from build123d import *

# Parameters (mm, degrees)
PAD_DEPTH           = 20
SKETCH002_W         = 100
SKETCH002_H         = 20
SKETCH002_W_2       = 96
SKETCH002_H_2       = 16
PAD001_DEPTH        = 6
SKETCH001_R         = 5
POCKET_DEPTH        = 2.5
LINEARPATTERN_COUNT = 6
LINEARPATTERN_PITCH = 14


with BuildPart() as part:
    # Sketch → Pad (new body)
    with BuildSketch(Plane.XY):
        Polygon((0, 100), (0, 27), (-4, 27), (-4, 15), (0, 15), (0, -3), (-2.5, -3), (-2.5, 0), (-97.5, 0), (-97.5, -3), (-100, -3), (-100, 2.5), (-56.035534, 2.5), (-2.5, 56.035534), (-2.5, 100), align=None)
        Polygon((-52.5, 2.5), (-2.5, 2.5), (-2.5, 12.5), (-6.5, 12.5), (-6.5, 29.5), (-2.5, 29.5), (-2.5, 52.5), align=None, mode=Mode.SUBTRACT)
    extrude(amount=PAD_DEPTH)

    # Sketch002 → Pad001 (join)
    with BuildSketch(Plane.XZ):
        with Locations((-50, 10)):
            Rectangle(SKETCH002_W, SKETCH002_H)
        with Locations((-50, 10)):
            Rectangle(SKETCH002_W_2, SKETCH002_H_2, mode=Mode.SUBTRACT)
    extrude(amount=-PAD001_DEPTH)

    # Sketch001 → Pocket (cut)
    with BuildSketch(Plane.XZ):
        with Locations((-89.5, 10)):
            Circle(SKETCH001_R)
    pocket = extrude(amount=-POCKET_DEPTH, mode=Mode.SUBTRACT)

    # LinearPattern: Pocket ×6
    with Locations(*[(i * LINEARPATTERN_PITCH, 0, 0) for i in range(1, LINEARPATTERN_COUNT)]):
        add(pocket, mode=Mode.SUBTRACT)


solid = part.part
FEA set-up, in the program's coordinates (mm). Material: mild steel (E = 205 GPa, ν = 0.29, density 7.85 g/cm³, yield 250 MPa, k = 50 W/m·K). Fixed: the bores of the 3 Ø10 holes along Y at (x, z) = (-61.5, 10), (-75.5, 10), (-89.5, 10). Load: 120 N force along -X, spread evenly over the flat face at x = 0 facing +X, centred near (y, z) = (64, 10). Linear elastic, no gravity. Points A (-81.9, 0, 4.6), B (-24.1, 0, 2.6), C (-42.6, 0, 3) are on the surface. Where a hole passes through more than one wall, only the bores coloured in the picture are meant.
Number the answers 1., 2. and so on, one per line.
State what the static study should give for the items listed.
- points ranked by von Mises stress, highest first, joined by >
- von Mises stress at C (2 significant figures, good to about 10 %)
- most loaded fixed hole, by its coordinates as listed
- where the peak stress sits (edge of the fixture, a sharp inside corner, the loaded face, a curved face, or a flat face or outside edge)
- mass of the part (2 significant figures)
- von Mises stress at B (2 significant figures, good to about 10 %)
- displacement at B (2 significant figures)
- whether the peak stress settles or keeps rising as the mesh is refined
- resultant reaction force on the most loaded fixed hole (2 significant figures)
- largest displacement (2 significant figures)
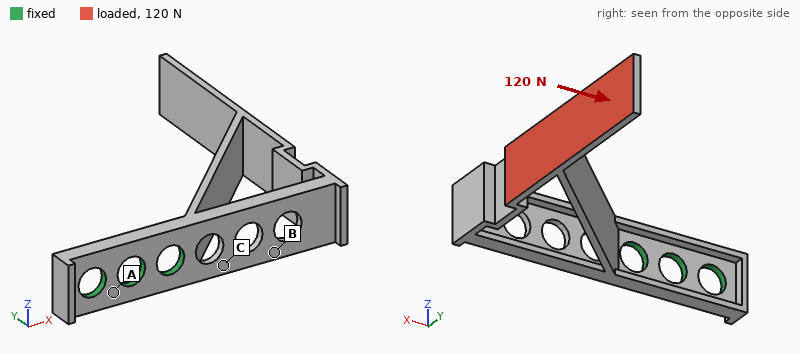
1. C > B > A
2. 89 MPa
3. (-75.5, 10)
4. edge of the fixture
5. 110 g
6. 42 MPa
7. 0.15 mm
8. keeps rising
9. 330 N
10. 0.88 mm
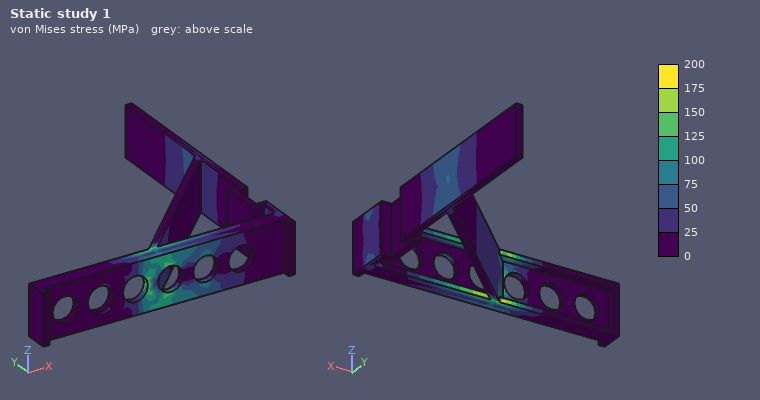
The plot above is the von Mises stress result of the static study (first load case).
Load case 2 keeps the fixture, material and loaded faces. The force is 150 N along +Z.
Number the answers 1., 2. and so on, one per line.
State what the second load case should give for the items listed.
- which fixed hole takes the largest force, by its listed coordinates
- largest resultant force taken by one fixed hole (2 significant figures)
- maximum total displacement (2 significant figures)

1. (-61.5, 10)
2. 250 N
3. 0.25 mm
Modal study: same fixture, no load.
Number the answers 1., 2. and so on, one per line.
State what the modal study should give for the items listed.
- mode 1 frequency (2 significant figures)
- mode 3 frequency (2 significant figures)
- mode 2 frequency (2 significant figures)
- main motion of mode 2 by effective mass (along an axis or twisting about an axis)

1. 320 Hz
2. 900 Hz
3. 800 Hz
4. along Z
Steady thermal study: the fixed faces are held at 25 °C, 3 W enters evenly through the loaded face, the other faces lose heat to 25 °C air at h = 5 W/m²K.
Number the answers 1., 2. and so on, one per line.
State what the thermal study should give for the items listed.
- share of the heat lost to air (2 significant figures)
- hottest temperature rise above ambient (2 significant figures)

1. 38 %
2. 53 K
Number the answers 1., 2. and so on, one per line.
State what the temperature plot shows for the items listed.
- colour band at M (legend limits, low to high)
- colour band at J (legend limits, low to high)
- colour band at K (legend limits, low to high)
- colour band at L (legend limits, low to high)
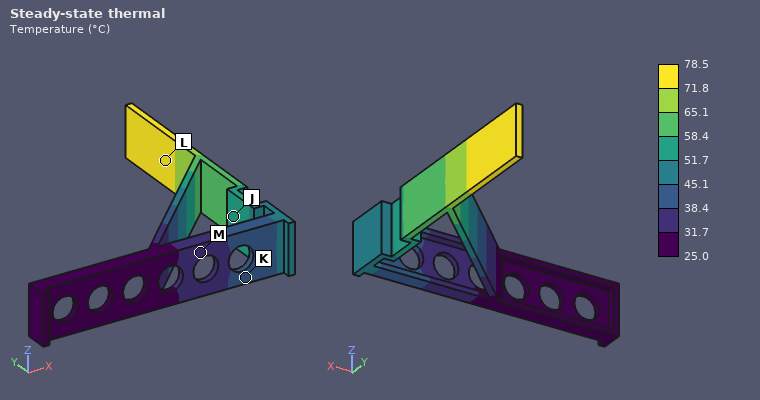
1. 31.7 to 38.4 °C
2. 51.7 to 58.4 °C
3. 38.4 to 45.1 °C
4. 71.8 to 78.5 °C
